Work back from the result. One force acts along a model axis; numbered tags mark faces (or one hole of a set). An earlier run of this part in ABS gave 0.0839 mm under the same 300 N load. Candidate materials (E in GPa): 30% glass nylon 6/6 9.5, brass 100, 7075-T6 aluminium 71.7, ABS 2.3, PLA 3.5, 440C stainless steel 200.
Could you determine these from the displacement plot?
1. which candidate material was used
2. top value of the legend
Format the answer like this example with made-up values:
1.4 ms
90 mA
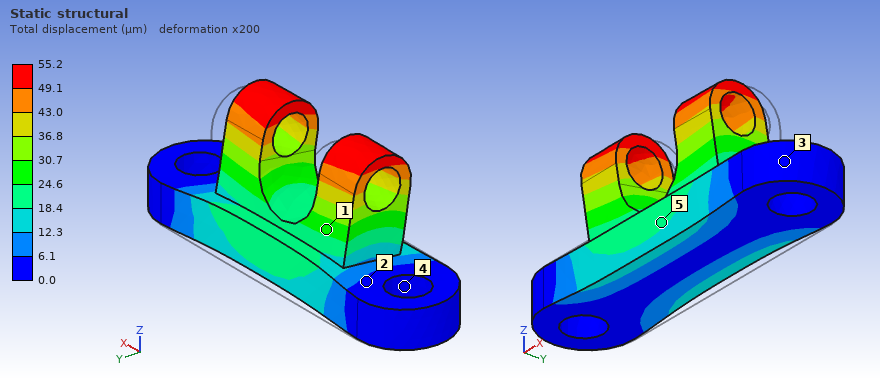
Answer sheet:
PLA
55.2 µm
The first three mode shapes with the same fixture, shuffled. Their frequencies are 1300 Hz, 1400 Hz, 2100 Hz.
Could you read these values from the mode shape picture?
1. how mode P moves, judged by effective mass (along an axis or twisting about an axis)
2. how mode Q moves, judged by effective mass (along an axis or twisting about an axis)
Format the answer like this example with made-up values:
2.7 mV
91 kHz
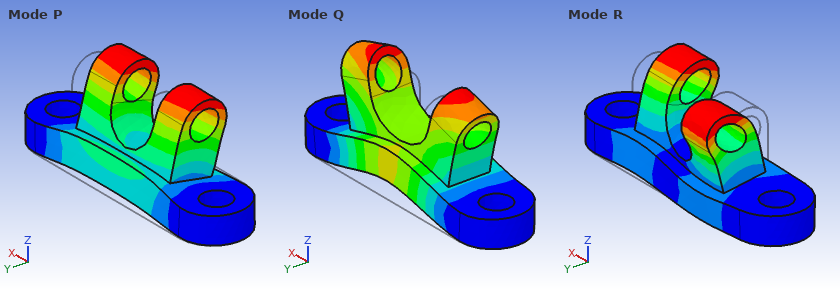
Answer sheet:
along Y
along Z
